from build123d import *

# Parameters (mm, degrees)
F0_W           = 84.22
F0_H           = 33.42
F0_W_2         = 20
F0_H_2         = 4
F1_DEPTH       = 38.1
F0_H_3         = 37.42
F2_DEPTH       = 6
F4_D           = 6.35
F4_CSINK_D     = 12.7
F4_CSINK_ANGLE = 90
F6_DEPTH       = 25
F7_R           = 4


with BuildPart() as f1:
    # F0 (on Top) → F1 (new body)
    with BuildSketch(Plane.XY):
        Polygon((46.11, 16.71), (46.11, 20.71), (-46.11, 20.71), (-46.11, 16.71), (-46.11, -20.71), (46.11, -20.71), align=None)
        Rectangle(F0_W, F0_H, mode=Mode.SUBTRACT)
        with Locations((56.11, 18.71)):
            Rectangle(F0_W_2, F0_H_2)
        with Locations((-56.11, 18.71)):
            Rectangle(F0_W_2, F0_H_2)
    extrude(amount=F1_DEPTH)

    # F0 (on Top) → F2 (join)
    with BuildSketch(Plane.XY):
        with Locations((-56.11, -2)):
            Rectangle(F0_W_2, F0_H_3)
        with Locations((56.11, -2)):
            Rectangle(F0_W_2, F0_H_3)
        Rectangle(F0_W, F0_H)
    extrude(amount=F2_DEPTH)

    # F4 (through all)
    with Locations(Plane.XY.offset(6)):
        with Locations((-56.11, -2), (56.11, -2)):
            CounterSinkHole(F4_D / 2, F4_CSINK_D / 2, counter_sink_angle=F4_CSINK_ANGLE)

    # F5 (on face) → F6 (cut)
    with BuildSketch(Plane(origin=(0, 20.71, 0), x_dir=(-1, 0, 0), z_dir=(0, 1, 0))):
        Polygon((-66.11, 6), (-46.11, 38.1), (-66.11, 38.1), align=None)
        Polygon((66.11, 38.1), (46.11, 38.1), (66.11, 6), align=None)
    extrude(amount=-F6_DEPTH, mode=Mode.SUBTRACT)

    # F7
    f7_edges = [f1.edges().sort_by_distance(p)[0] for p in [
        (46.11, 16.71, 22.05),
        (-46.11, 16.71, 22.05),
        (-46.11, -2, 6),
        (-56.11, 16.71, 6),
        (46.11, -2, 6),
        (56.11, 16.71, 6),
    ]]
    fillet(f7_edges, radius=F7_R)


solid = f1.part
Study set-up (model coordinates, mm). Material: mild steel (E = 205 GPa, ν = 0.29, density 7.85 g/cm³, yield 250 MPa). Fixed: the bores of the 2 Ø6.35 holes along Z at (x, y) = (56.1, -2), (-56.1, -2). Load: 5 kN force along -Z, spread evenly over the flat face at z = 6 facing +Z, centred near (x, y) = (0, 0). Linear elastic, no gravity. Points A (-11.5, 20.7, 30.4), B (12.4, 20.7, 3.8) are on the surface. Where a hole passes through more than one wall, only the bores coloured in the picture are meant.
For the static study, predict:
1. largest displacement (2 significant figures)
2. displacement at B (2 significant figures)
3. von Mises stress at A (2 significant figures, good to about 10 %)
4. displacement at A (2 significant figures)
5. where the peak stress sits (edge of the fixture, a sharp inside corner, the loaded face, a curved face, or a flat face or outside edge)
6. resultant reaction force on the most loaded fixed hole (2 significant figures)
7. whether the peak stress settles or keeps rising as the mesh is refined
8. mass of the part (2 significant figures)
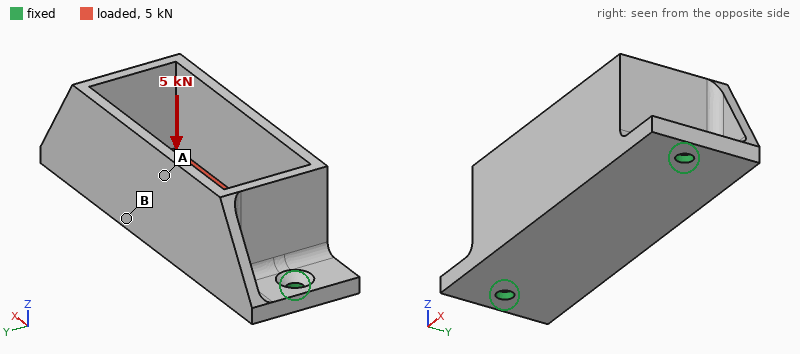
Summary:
27 µm
25 µm
23 MPa
25 µm
edge of the fixture
3.2 kN
keeps rising
530 g
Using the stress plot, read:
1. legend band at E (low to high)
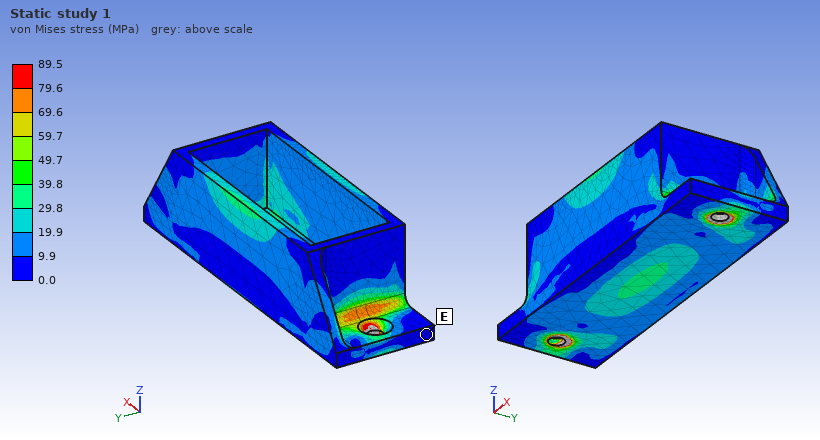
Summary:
0.0 to 9.9 MPa
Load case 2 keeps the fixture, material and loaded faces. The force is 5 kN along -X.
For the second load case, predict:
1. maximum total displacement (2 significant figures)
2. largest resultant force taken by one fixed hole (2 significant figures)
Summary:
3.0 µm
2.5 kN
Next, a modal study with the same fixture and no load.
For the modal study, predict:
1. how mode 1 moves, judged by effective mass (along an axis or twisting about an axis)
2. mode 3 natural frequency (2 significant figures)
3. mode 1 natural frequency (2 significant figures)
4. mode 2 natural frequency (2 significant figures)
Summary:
along Y
3900 Hz
1400 Hz
3000 Hz
